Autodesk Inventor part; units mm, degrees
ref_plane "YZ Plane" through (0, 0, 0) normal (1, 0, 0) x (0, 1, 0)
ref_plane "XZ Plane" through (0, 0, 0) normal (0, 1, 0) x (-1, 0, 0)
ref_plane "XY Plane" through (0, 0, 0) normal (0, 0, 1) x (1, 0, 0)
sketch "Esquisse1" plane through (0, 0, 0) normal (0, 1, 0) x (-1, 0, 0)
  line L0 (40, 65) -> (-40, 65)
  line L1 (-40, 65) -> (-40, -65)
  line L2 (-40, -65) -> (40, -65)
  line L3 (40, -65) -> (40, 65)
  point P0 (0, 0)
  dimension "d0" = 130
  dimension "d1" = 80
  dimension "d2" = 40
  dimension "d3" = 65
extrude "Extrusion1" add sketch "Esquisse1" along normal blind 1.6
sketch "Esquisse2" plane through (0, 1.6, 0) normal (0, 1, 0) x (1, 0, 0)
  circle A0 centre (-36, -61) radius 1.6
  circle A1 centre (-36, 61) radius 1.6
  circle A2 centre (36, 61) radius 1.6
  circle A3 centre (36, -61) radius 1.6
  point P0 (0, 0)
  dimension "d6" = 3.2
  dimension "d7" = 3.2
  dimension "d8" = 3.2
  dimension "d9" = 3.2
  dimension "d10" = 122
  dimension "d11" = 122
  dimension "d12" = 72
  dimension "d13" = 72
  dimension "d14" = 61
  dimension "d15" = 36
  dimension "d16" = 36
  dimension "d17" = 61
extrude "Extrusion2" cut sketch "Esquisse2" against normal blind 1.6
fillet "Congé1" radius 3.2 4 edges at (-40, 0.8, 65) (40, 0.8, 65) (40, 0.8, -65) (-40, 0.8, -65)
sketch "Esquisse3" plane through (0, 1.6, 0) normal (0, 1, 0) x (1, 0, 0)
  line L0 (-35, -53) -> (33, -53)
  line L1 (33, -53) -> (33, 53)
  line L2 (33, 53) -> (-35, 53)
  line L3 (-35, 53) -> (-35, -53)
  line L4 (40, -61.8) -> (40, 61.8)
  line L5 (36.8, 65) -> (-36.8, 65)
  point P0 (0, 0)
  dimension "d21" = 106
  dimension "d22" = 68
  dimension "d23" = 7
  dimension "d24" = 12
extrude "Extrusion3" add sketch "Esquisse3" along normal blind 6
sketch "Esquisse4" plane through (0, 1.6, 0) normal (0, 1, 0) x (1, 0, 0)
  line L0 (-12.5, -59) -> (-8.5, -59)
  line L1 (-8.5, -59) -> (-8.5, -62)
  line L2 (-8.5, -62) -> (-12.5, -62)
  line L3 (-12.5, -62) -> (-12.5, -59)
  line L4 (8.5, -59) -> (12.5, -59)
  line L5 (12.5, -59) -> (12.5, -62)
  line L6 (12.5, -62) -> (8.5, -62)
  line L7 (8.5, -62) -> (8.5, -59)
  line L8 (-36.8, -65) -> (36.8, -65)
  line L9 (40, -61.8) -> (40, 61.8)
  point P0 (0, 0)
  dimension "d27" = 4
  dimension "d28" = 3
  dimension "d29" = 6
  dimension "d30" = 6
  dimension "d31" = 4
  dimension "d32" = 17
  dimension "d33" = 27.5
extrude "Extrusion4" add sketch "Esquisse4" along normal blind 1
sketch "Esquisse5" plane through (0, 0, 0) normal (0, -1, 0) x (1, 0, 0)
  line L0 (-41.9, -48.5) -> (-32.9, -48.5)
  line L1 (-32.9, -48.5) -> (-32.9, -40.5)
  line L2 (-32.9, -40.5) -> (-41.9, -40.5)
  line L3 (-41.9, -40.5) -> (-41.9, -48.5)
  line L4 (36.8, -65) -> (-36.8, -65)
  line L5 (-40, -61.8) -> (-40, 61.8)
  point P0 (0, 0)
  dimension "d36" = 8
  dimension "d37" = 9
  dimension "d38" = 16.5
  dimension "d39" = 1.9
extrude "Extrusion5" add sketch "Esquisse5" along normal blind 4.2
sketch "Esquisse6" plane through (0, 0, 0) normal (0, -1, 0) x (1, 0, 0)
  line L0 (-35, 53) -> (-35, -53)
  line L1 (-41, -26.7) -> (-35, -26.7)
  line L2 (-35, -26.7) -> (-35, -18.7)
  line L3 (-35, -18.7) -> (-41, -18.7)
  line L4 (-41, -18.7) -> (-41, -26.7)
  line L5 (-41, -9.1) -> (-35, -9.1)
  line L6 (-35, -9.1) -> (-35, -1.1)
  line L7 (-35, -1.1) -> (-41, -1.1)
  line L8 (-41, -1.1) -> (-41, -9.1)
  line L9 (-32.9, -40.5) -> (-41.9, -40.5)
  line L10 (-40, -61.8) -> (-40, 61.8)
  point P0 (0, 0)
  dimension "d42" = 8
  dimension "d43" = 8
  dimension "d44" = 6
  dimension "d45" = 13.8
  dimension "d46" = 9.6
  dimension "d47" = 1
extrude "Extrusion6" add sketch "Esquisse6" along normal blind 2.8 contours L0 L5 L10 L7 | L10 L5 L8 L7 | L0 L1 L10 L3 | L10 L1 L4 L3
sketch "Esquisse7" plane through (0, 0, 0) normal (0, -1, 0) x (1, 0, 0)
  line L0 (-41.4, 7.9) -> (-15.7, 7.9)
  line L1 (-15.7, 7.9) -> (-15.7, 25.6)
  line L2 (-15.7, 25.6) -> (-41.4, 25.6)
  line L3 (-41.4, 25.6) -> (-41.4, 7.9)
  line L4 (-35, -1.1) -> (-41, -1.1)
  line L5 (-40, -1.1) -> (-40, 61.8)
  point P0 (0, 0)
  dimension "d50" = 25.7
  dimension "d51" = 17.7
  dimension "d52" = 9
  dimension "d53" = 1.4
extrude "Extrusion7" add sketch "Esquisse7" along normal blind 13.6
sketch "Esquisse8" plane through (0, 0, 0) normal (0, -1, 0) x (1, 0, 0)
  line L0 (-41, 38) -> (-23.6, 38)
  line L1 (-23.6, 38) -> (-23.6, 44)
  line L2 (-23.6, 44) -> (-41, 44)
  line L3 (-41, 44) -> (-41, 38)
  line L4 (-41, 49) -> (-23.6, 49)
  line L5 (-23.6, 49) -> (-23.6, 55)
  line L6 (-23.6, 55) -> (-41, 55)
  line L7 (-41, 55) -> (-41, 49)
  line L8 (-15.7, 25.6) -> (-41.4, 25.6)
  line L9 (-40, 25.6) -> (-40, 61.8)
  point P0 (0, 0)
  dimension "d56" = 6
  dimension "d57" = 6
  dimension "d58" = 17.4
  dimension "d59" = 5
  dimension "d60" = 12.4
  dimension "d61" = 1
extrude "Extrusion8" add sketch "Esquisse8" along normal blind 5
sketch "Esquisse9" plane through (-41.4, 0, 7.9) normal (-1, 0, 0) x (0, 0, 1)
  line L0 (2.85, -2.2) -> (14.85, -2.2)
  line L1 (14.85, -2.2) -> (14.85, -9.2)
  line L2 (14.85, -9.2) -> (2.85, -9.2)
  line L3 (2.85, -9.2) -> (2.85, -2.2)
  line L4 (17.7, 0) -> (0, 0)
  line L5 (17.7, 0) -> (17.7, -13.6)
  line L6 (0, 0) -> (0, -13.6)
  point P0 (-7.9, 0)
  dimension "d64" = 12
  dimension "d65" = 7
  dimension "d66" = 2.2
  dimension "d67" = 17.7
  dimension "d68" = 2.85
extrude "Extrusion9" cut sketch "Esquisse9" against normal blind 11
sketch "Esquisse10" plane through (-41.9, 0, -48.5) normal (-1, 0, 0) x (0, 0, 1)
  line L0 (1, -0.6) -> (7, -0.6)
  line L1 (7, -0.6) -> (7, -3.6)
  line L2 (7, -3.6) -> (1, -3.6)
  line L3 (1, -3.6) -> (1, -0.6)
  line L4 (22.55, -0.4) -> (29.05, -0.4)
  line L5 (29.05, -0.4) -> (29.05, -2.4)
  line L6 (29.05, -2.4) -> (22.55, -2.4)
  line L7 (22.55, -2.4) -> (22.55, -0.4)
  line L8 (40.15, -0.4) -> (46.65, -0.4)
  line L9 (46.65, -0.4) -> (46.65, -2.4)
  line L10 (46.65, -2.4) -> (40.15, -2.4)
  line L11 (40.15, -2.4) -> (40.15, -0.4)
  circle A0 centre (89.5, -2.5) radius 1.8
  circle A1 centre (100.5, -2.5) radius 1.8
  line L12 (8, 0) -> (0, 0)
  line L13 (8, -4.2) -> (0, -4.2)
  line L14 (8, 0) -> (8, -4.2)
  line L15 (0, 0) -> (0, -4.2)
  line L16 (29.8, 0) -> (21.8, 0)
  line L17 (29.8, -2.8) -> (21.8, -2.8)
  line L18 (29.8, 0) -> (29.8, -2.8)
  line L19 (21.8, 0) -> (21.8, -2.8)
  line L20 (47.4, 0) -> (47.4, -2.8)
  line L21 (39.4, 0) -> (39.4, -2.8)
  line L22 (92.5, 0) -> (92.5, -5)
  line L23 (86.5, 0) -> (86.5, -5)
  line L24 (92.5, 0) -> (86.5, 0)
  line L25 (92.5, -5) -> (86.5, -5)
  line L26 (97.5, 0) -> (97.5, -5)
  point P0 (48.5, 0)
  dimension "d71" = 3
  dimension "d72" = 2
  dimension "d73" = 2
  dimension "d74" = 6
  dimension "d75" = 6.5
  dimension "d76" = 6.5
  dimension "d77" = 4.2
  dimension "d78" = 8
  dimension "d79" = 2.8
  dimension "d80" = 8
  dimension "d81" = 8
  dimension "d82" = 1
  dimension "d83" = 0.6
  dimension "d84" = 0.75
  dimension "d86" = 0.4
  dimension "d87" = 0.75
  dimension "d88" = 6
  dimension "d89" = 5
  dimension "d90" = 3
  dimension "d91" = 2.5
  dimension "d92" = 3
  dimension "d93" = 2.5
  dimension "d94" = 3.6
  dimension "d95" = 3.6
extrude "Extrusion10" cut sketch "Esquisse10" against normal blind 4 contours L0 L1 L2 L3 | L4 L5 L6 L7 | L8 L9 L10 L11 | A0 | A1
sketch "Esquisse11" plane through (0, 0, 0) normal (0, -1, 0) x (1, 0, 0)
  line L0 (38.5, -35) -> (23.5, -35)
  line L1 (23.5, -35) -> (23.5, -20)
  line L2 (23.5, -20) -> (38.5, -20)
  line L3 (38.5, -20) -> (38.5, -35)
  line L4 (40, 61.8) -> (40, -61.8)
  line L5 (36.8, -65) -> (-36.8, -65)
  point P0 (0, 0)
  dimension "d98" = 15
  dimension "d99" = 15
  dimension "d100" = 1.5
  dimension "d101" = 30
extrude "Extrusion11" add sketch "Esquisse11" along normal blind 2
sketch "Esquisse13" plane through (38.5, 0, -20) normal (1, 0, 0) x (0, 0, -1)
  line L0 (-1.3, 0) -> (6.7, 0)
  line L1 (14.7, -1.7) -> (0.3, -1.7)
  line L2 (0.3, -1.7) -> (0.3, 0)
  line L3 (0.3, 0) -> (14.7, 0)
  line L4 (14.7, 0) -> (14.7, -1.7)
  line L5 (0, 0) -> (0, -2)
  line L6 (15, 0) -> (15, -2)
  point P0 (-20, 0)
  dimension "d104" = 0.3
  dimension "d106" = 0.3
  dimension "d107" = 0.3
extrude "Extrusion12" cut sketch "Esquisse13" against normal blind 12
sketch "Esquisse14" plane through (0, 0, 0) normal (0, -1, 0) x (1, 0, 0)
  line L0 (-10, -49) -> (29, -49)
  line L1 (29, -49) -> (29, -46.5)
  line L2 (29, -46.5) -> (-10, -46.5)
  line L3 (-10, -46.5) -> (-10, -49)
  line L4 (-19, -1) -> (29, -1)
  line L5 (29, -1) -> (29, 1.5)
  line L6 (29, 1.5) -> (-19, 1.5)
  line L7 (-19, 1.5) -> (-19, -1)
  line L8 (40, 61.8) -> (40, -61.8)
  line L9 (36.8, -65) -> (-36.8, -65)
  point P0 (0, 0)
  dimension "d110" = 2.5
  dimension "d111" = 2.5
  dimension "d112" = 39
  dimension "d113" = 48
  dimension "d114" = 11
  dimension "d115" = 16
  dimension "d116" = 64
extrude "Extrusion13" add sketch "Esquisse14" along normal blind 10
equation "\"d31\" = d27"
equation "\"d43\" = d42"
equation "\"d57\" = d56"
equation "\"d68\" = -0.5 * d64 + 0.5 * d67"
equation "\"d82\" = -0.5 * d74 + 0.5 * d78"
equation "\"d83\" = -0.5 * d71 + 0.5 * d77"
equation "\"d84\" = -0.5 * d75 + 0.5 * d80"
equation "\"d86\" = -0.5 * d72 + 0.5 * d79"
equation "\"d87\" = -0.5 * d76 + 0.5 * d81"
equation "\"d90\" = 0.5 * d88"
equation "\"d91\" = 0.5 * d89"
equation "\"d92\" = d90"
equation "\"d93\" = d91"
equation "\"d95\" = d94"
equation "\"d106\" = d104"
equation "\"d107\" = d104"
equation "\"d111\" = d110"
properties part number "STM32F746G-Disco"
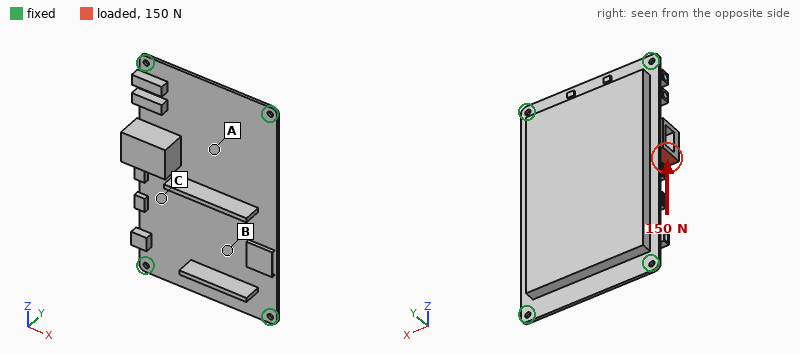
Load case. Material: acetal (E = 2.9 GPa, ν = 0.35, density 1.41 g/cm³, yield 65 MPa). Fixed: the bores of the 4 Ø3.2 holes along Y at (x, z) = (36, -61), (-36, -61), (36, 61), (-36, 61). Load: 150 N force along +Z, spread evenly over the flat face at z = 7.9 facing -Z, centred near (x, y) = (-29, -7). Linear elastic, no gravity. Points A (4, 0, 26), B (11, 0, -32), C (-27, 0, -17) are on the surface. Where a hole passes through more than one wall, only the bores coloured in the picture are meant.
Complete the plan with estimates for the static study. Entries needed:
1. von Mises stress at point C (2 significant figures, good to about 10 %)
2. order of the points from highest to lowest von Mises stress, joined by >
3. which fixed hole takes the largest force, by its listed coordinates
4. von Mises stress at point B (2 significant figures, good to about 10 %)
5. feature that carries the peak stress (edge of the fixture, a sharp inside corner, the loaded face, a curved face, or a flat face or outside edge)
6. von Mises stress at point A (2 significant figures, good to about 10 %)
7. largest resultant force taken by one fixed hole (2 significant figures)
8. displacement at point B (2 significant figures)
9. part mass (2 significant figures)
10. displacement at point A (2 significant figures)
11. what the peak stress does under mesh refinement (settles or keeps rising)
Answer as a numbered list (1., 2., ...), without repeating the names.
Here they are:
1. 1.2 MPa
2. C > A > B
3. (-36, 61)
4. 0.40 MPa
5. edge of the fixture
6. 0.66 MPa
7. 66 N
8. 0.055 mm
9. 97 g
10. 0.023 mm
11. keeps rising
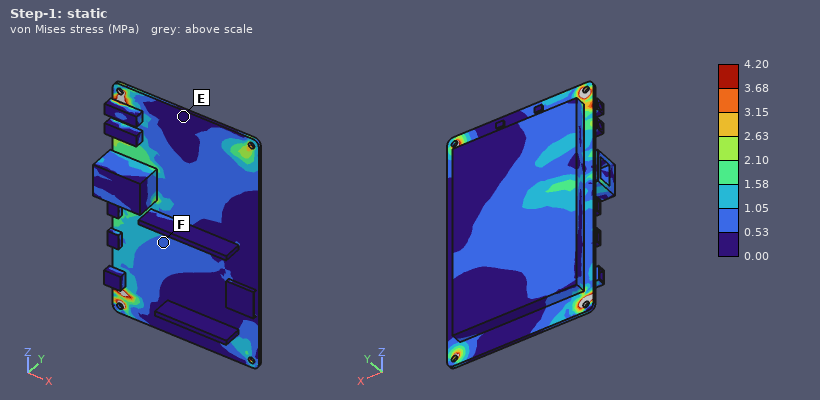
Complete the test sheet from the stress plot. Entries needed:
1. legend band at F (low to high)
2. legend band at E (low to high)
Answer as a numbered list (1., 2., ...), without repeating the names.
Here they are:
1. 0.53 to 1.05 MPa
2. 0.00 to 0.53 MPa
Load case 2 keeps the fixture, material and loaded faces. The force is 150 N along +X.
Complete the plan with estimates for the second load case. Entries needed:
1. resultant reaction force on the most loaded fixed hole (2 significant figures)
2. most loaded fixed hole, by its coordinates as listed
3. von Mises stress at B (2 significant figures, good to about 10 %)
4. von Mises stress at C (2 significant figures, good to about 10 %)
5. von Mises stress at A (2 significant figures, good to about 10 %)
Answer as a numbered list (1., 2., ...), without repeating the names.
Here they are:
1. 50 N
2. (-36, 61)
3. 0.99 MPa
4. 1.3 MPa
5. 1.2 MPa
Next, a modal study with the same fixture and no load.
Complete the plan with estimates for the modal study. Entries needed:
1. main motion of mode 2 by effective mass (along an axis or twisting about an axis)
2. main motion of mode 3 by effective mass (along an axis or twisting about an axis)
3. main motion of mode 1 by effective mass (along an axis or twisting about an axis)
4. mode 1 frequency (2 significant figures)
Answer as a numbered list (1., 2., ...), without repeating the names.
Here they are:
1. twisting about Z
2. twisting about X
3. along Y
4. 310 Hz
